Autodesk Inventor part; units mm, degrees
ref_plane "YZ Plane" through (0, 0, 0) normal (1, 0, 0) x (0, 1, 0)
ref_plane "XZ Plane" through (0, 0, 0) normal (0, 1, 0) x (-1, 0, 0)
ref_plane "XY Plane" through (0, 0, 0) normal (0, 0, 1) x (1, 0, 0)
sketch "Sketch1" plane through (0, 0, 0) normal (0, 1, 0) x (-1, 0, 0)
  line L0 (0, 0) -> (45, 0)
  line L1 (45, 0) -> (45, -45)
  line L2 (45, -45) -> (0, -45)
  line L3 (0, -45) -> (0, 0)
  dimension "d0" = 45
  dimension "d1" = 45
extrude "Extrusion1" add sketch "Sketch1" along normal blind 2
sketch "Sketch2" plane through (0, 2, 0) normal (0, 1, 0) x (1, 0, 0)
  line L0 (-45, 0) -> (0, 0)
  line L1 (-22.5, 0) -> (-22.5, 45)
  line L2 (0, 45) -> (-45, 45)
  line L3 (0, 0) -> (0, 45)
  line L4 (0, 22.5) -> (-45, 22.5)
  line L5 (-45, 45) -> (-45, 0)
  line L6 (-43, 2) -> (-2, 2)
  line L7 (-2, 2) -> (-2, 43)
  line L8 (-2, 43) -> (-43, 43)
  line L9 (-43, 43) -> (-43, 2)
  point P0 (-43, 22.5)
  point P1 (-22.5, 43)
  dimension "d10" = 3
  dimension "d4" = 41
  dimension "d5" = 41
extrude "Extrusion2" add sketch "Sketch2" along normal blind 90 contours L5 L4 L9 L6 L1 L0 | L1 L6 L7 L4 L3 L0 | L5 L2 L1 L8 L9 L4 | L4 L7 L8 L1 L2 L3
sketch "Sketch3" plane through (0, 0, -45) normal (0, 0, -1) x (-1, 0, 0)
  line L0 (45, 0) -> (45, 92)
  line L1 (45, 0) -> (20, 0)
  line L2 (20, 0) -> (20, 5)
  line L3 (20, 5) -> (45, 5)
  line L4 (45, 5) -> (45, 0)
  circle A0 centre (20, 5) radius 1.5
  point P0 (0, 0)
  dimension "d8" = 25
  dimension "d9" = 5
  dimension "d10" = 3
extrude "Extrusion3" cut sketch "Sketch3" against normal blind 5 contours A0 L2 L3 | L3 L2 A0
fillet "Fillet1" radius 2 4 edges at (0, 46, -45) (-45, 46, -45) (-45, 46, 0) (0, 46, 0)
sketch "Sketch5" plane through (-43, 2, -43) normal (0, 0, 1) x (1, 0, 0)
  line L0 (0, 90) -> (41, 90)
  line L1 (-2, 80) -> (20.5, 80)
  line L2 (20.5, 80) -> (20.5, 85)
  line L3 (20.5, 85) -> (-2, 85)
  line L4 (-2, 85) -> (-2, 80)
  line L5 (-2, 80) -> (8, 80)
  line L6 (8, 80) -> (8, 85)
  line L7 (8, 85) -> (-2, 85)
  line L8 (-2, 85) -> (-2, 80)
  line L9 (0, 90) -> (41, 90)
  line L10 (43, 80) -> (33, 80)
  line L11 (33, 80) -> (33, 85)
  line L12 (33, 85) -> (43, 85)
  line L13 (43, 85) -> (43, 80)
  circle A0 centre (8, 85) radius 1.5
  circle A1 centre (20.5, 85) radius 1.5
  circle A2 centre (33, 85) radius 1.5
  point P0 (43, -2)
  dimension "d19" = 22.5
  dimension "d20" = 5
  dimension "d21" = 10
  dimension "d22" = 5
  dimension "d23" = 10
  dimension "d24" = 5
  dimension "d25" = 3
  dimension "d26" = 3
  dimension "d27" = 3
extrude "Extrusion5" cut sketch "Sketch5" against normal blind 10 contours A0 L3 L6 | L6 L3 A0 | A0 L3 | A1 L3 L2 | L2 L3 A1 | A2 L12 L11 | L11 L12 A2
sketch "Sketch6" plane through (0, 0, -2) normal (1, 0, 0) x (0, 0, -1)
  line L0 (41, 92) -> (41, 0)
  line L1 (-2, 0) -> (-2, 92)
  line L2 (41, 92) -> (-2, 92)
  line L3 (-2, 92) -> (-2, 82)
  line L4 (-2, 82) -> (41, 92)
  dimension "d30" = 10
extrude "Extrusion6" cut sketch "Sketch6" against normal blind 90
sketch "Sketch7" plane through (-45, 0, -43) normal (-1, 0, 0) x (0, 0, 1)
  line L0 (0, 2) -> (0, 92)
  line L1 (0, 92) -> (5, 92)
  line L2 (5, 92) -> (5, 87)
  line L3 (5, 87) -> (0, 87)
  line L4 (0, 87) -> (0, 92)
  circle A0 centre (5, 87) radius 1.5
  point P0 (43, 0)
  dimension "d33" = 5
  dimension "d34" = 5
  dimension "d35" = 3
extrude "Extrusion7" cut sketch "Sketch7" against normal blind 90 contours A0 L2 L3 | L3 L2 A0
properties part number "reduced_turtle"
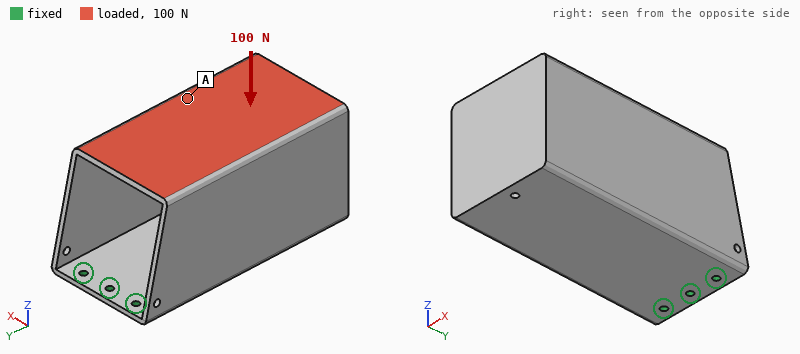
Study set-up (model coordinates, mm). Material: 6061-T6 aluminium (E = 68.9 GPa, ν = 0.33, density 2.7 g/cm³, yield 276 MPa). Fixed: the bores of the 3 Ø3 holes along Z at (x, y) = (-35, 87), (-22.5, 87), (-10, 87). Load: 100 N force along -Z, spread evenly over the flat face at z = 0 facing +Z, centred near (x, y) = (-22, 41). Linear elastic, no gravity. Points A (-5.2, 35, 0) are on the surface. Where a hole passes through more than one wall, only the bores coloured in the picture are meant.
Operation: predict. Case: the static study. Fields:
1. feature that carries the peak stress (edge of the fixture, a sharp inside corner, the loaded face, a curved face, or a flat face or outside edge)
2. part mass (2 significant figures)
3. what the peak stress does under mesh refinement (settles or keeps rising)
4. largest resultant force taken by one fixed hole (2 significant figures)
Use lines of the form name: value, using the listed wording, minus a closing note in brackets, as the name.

feature that carries the peak stress: edge of the fixture
part mass: 89 g
what the peak stress does under mesh refinement: keeps rising
largest resultant force taken by one fixed hole: 43 N
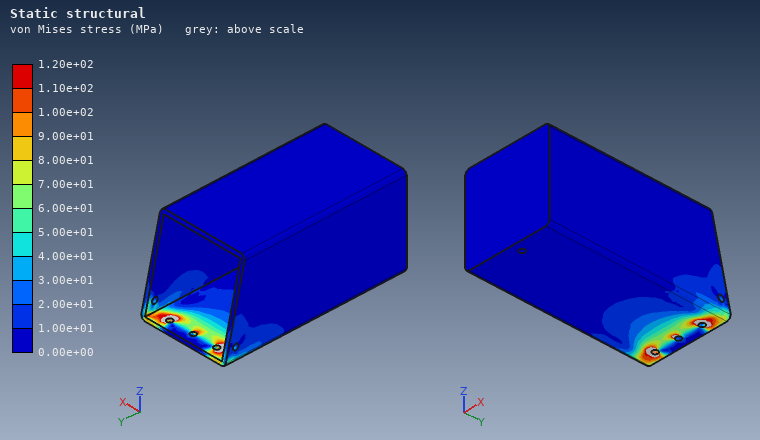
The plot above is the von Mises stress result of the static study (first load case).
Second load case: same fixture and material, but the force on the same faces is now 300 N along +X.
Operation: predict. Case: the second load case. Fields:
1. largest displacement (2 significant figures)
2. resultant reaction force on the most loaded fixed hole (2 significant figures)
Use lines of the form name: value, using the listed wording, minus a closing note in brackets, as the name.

largest displacement: 1.2 mm
resultant reaction force on the most loaded fixed hole: 610 N
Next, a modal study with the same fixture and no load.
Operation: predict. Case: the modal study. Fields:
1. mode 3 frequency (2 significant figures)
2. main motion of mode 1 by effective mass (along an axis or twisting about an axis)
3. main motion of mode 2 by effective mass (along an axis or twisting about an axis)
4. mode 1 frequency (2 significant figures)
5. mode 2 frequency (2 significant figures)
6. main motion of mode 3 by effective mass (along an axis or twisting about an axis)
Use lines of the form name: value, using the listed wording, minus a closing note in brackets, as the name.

mode 3 frequency: 1900 Hz
main motion of mode 1 by effective mass: along Z
main motion of mode 2 by effective mass: along X
mode 1 frequency: 180 Hz
mode 2 frequency: 450 Hz
main motion of mode 3 by effective mass: along X
